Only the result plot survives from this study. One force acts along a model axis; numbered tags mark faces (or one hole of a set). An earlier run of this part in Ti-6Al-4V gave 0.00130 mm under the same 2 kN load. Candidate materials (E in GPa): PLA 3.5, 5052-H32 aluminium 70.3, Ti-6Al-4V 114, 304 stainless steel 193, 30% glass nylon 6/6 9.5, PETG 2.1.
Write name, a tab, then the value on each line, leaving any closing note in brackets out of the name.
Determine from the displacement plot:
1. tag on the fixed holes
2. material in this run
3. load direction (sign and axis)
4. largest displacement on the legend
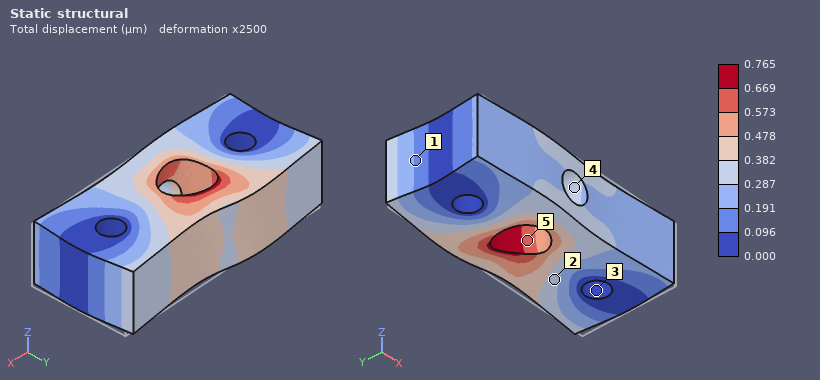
tag on the fixed holes	3
material in this run	304 stainless steel
load direction	-X
largest displacement on the legend	0.765 µm
